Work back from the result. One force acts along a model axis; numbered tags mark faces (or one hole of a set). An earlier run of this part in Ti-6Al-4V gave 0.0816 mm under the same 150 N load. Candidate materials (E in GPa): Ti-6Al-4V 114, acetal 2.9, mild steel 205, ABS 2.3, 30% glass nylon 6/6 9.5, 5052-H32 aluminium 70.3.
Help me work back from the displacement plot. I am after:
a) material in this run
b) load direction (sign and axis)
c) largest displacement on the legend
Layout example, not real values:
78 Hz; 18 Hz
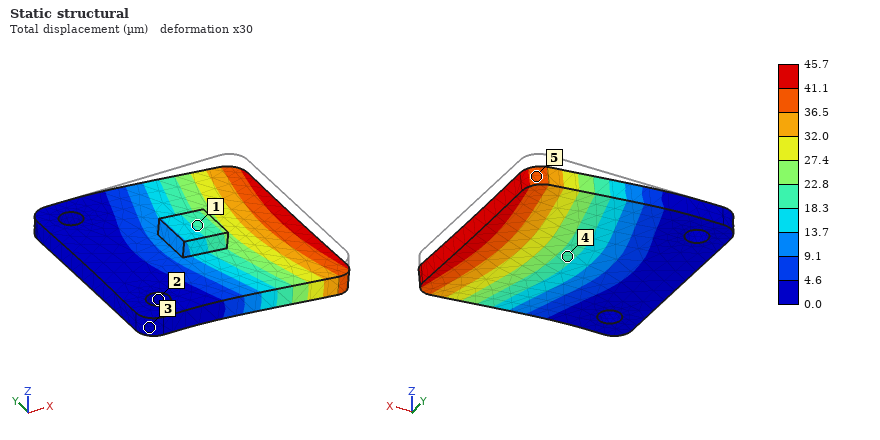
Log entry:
mild steel; -Z; 45.7 µm
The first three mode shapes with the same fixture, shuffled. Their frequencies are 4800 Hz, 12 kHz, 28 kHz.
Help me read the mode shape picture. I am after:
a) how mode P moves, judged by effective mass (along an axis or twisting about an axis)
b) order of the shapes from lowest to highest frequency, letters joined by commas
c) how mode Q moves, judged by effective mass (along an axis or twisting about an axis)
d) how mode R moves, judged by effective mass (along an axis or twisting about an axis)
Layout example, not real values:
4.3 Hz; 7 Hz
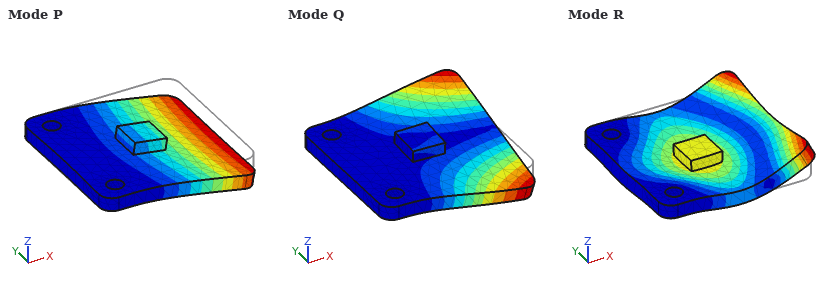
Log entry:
along Z; P, Q, R; twisting about X; along Z
